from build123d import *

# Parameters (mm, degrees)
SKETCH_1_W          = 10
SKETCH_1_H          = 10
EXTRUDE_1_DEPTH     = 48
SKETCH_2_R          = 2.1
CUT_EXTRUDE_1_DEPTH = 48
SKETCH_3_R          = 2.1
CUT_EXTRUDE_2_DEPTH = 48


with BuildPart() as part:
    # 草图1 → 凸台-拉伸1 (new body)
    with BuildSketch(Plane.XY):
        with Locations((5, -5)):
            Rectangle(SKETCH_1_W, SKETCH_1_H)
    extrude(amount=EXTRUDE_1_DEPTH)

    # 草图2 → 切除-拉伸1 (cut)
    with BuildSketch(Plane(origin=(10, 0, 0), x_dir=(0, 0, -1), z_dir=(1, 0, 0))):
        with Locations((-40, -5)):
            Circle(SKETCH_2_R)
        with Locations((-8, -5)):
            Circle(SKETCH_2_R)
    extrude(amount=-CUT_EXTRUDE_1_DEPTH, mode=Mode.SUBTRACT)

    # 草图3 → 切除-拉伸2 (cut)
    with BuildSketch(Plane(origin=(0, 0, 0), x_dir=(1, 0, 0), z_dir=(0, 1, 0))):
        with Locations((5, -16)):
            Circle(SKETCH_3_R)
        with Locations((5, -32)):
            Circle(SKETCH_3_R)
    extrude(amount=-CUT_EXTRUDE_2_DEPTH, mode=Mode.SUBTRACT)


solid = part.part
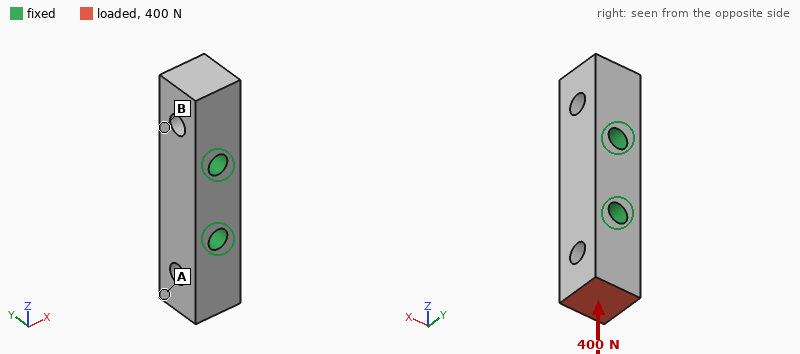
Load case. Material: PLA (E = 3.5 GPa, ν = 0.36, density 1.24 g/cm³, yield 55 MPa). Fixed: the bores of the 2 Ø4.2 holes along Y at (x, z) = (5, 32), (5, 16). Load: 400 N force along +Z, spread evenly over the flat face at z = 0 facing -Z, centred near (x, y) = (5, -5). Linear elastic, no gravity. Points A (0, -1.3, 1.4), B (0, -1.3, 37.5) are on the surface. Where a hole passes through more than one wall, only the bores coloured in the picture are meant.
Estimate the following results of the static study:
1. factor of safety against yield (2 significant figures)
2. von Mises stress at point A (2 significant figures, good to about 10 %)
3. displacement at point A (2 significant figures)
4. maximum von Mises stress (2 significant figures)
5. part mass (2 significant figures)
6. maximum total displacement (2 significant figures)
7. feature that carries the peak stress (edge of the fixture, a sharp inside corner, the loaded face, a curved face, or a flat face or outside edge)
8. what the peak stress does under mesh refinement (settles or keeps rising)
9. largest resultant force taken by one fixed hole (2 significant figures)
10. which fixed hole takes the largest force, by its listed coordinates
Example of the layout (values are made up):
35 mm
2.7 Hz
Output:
3.7
4.3 MPa
22 µm
15 MPa
5.3 g
25 µm
a curved face
settles
380 N
(5, 16)
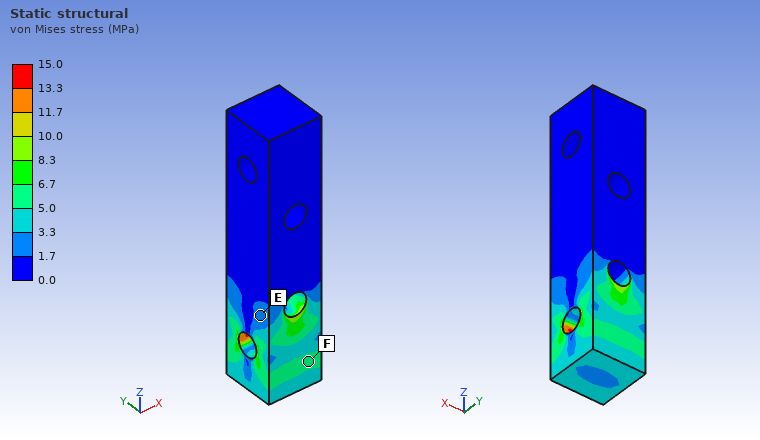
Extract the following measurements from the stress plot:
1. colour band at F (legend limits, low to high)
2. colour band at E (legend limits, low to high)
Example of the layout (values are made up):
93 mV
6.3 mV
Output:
5.0 to 6.7 MPa
1.7 to 3.3 MPa
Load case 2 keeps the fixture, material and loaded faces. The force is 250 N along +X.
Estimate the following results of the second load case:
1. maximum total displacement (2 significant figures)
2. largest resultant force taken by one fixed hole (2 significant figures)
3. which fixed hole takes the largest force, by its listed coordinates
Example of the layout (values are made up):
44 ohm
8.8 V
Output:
0.23 mm
320 N
(5, 16)
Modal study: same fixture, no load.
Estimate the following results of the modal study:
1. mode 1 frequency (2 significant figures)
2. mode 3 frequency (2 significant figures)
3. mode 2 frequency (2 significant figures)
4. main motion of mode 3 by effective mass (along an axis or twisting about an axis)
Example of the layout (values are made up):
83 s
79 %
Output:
7400 Hz
8400 Hz
7400 Hz
along Y
